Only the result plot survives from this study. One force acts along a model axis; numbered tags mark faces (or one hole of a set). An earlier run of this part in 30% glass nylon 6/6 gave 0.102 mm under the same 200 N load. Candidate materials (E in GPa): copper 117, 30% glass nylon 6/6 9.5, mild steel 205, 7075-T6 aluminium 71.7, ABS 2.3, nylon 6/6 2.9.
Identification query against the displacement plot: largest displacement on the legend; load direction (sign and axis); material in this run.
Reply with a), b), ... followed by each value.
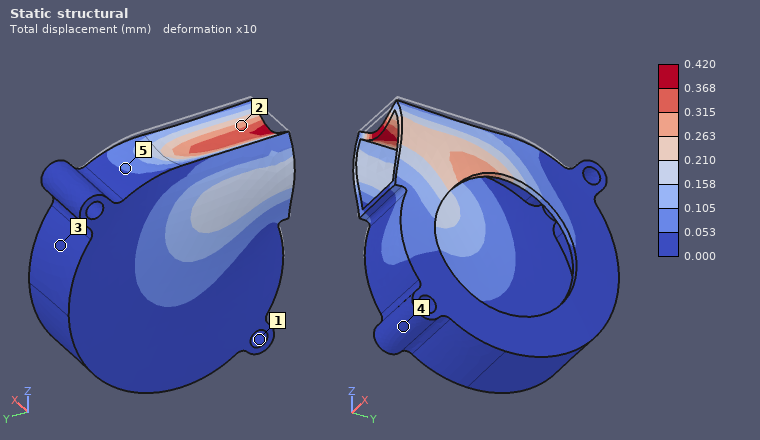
a) 0.420 mm
b) -Z
c) ABS
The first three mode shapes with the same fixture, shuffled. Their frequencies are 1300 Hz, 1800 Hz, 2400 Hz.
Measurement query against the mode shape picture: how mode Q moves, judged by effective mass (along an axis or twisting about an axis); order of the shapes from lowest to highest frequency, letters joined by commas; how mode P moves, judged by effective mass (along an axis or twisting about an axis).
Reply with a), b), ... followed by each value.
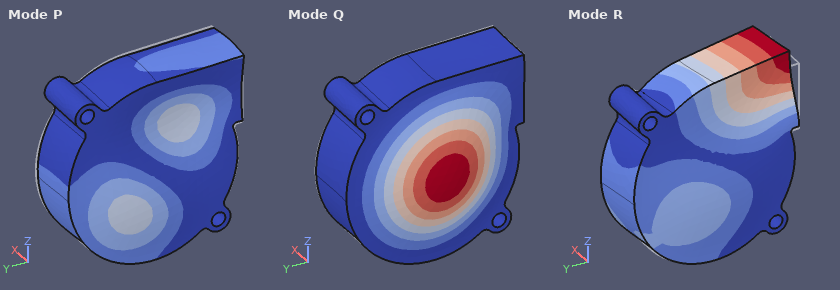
a) along X
b) Q, R, P
c) along X
